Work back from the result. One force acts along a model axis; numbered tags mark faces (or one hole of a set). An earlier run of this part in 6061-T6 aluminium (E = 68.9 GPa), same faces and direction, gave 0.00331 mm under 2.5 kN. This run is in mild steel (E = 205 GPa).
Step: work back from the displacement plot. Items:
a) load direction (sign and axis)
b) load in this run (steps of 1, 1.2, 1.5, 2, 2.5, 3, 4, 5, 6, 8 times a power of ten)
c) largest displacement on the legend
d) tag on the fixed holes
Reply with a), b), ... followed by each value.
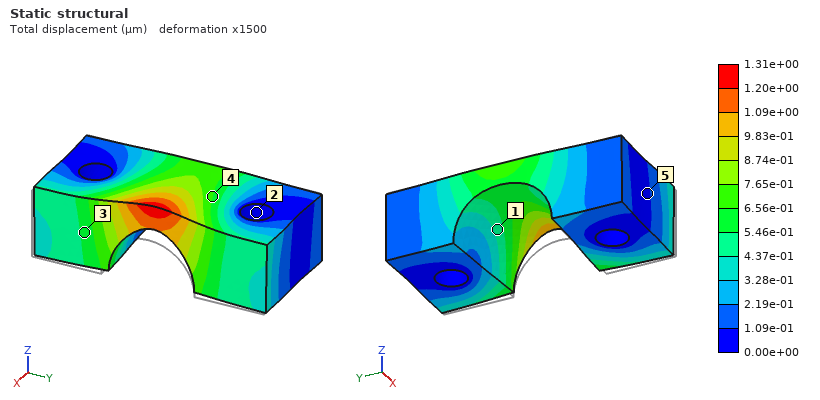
a) -X
b) 3 kN
c) 1.31e+00 µm
d) 2
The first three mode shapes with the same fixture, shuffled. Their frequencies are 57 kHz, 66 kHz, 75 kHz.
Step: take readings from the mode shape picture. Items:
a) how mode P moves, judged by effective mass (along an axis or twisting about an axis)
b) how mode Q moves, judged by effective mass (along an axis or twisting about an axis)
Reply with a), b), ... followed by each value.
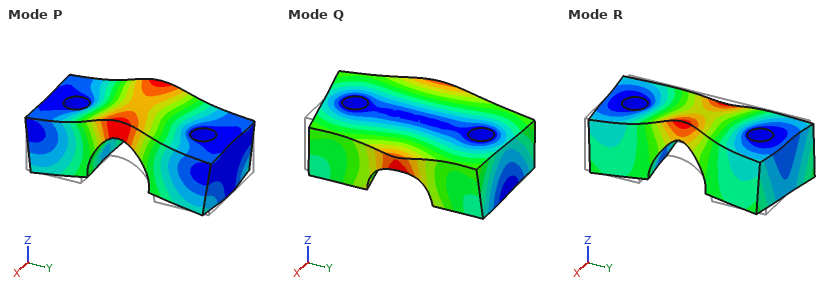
a) along Z
b) twisting about Y
